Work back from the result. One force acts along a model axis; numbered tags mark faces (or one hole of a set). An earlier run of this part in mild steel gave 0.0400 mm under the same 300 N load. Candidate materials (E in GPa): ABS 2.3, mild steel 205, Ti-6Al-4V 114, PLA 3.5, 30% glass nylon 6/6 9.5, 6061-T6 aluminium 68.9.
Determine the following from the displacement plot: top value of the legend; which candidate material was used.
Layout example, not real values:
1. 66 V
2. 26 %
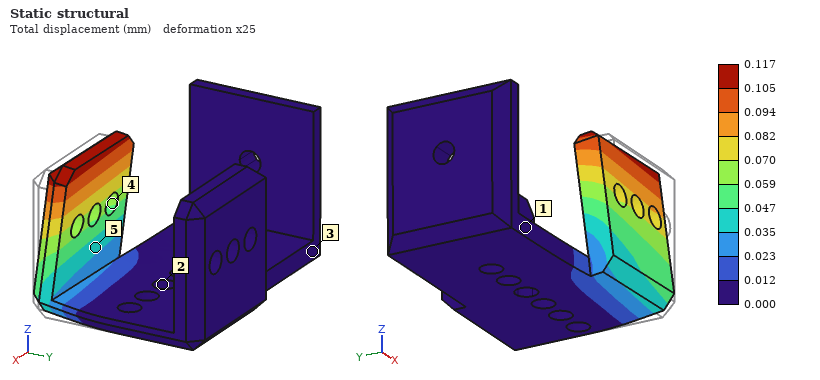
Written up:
1. 0.117 mm
2. 6061-T6 aluminium
